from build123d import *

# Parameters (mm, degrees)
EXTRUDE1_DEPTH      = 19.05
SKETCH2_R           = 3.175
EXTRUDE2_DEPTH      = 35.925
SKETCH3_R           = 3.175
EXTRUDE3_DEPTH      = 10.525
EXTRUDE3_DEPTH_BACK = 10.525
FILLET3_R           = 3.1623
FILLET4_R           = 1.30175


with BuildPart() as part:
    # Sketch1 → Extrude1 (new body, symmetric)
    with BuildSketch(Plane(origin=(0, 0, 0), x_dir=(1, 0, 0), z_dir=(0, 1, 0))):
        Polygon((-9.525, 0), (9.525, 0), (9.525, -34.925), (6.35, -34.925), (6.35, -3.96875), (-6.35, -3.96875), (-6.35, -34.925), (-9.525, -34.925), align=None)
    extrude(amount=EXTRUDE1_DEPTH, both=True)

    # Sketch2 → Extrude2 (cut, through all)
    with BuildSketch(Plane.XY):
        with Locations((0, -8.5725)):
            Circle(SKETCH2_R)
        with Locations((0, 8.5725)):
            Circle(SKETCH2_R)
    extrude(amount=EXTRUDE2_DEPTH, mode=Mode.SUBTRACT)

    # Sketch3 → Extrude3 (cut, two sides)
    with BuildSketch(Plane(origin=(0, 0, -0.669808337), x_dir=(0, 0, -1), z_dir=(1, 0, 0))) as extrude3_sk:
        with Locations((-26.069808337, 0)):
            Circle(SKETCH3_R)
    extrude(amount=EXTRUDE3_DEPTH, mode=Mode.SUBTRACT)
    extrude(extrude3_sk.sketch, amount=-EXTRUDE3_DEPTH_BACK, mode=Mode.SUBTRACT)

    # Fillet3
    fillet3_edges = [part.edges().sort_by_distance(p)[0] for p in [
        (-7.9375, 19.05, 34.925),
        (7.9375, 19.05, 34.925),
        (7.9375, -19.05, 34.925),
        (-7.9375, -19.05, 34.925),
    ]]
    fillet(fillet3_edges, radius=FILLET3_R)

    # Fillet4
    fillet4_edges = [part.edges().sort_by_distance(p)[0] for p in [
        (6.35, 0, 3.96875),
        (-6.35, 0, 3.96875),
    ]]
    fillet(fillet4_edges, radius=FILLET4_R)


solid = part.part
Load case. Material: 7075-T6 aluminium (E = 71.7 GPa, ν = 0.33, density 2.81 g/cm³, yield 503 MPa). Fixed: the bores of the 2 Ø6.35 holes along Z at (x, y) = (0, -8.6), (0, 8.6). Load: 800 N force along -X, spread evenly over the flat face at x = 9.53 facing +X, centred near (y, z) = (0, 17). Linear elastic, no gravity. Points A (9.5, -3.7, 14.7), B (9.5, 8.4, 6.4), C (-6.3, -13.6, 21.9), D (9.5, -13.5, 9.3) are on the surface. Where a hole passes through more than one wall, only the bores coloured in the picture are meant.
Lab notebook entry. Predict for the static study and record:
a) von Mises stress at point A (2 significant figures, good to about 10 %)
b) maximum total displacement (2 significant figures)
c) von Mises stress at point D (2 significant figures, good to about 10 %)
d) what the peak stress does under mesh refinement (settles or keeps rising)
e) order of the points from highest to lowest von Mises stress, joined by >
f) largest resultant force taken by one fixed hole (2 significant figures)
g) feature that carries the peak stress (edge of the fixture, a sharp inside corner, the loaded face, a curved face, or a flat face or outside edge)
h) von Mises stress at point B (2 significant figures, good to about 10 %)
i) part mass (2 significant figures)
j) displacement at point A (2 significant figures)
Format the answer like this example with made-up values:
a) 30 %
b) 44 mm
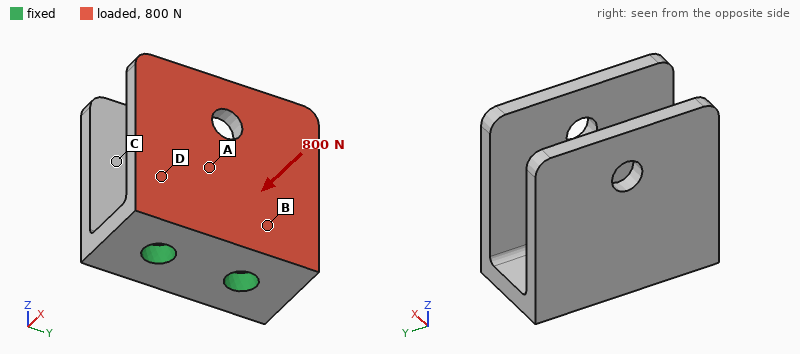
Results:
a) 62 MPa
b) 0.51 mm
c) 100 MPa
d) keeps rising
e) B > D > A > C
f) 400 N
g) edge of the fixture
h) 130 MPa
i) 28 g
j) 0.14 mm
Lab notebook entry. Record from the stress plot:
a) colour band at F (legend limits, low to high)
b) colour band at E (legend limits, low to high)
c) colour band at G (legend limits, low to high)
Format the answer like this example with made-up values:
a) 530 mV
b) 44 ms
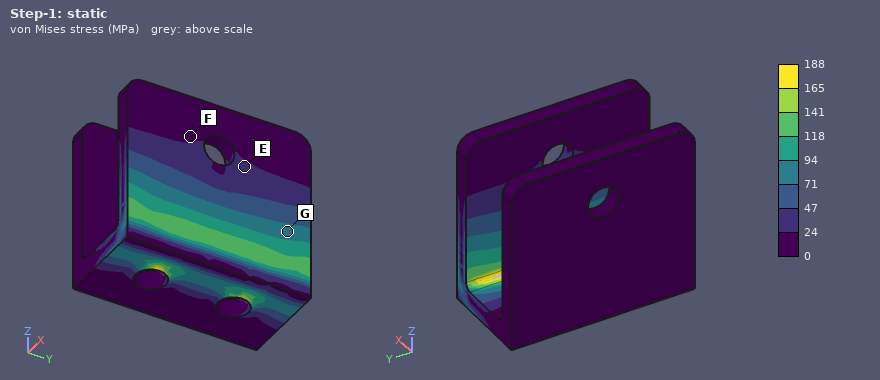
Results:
a) 0 to 24 MPa
b) 24 to 47 MPa
c) 71 to 94 MPa
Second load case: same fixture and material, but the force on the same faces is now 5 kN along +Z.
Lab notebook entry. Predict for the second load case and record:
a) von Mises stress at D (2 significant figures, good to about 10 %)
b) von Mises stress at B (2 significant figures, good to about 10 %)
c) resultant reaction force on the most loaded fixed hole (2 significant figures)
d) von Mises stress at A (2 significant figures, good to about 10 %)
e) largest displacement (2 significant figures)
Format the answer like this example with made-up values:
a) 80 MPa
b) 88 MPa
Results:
a) 110 MPa
b) 140 MPa
c) 2.5 kN
d) 87 MPa
e) 0.66 mm
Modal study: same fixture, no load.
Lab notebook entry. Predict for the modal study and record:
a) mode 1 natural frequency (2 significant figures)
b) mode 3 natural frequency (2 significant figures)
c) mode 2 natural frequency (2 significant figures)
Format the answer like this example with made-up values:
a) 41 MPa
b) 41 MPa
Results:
a) 2300 Hz
b) 4800 Hz
c) 2300 Hz
